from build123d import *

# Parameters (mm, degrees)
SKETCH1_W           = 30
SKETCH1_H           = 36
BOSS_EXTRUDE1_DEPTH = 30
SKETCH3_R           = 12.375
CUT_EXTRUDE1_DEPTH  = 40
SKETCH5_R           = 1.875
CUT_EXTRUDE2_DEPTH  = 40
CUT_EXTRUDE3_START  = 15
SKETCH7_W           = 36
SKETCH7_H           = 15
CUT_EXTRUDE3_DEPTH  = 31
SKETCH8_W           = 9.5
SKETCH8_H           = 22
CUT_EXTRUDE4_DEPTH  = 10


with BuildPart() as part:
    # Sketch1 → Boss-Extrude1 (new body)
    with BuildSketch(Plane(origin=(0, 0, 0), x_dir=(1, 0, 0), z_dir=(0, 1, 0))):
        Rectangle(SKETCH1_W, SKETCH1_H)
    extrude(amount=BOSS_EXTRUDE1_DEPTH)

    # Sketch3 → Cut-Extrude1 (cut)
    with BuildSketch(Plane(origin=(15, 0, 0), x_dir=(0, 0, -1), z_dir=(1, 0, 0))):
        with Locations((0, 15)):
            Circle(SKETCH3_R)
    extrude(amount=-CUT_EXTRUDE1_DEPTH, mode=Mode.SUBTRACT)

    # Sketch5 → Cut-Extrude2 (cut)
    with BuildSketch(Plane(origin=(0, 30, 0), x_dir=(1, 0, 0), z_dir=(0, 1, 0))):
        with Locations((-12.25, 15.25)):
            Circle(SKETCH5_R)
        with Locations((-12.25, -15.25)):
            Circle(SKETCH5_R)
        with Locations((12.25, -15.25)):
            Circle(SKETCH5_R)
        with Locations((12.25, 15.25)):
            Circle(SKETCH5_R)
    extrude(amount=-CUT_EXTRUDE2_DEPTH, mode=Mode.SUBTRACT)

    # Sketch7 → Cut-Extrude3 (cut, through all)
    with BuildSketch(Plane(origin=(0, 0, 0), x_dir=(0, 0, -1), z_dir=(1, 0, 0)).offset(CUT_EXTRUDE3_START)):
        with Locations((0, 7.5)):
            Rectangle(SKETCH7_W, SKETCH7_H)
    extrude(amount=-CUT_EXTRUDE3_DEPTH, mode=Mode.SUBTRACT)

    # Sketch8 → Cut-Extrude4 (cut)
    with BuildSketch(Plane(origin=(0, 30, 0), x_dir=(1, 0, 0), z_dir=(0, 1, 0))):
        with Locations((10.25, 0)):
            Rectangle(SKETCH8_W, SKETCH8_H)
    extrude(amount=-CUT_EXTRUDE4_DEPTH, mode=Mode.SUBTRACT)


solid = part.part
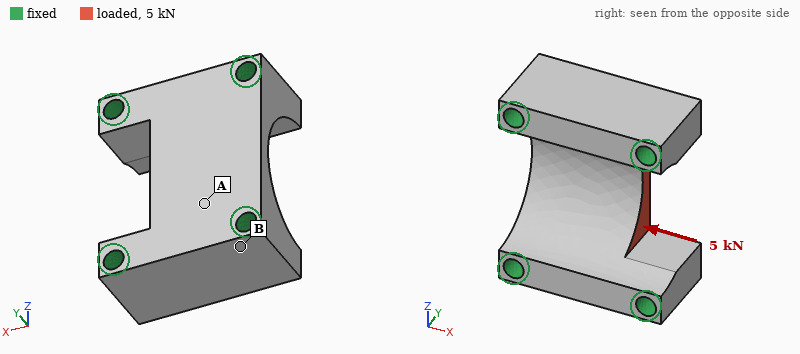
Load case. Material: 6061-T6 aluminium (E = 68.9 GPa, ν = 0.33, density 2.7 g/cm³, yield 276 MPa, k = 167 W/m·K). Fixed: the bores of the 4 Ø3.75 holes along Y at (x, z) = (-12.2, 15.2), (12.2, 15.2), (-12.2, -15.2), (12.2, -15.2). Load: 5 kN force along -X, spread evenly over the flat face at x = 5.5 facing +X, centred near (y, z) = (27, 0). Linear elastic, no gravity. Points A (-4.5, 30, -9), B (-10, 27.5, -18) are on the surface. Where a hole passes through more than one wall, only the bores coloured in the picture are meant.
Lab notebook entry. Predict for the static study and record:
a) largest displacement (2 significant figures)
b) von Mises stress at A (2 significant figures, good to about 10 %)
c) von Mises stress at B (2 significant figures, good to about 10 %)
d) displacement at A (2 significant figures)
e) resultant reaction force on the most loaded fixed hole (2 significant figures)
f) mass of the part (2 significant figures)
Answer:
16 µm
38 MPa
9.6 MPa
4.6 µm
1.7 kN
20 g
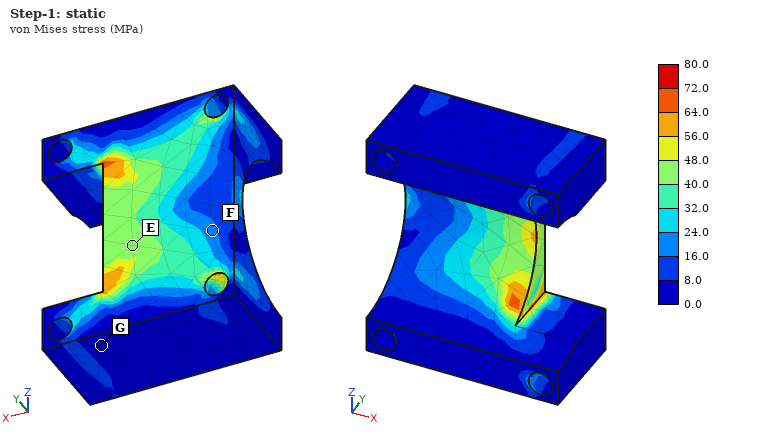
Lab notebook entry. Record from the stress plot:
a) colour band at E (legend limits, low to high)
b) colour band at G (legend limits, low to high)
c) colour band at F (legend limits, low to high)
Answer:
40.0 to 48.0 MPa
0.0 to 8.0 MPa
16.0 to 24.0 MPa
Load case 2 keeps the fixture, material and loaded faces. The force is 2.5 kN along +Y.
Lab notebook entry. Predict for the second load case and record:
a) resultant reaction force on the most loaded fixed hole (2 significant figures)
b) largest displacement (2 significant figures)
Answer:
1000 N
44 µm
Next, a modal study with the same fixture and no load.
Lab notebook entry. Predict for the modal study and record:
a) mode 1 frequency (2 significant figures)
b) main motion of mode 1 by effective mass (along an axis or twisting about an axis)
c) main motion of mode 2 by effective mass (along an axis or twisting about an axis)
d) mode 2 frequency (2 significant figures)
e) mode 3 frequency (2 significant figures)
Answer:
36 kHz
along Y
along Z
45 kHz
49 kHz
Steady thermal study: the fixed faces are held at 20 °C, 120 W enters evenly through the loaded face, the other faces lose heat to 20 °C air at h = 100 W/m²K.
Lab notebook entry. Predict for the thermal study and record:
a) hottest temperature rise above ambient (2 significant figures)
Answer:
67 K
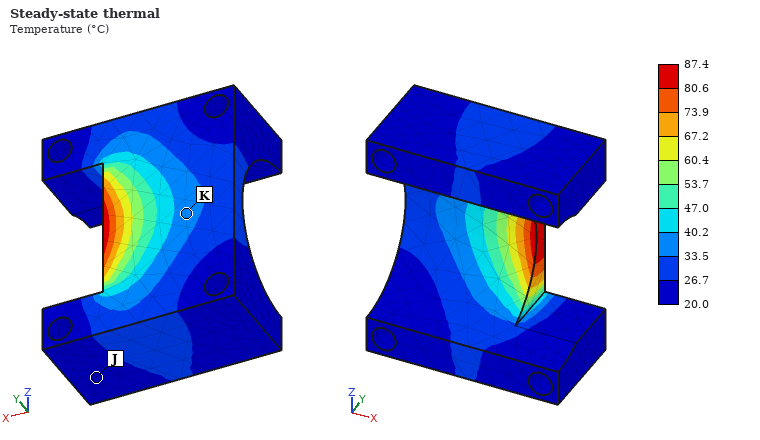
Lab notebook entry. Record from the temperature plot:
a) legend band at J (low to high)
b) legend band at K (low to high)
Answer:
20.0 to 26.7 °C
33.5 to 40.2 °C
